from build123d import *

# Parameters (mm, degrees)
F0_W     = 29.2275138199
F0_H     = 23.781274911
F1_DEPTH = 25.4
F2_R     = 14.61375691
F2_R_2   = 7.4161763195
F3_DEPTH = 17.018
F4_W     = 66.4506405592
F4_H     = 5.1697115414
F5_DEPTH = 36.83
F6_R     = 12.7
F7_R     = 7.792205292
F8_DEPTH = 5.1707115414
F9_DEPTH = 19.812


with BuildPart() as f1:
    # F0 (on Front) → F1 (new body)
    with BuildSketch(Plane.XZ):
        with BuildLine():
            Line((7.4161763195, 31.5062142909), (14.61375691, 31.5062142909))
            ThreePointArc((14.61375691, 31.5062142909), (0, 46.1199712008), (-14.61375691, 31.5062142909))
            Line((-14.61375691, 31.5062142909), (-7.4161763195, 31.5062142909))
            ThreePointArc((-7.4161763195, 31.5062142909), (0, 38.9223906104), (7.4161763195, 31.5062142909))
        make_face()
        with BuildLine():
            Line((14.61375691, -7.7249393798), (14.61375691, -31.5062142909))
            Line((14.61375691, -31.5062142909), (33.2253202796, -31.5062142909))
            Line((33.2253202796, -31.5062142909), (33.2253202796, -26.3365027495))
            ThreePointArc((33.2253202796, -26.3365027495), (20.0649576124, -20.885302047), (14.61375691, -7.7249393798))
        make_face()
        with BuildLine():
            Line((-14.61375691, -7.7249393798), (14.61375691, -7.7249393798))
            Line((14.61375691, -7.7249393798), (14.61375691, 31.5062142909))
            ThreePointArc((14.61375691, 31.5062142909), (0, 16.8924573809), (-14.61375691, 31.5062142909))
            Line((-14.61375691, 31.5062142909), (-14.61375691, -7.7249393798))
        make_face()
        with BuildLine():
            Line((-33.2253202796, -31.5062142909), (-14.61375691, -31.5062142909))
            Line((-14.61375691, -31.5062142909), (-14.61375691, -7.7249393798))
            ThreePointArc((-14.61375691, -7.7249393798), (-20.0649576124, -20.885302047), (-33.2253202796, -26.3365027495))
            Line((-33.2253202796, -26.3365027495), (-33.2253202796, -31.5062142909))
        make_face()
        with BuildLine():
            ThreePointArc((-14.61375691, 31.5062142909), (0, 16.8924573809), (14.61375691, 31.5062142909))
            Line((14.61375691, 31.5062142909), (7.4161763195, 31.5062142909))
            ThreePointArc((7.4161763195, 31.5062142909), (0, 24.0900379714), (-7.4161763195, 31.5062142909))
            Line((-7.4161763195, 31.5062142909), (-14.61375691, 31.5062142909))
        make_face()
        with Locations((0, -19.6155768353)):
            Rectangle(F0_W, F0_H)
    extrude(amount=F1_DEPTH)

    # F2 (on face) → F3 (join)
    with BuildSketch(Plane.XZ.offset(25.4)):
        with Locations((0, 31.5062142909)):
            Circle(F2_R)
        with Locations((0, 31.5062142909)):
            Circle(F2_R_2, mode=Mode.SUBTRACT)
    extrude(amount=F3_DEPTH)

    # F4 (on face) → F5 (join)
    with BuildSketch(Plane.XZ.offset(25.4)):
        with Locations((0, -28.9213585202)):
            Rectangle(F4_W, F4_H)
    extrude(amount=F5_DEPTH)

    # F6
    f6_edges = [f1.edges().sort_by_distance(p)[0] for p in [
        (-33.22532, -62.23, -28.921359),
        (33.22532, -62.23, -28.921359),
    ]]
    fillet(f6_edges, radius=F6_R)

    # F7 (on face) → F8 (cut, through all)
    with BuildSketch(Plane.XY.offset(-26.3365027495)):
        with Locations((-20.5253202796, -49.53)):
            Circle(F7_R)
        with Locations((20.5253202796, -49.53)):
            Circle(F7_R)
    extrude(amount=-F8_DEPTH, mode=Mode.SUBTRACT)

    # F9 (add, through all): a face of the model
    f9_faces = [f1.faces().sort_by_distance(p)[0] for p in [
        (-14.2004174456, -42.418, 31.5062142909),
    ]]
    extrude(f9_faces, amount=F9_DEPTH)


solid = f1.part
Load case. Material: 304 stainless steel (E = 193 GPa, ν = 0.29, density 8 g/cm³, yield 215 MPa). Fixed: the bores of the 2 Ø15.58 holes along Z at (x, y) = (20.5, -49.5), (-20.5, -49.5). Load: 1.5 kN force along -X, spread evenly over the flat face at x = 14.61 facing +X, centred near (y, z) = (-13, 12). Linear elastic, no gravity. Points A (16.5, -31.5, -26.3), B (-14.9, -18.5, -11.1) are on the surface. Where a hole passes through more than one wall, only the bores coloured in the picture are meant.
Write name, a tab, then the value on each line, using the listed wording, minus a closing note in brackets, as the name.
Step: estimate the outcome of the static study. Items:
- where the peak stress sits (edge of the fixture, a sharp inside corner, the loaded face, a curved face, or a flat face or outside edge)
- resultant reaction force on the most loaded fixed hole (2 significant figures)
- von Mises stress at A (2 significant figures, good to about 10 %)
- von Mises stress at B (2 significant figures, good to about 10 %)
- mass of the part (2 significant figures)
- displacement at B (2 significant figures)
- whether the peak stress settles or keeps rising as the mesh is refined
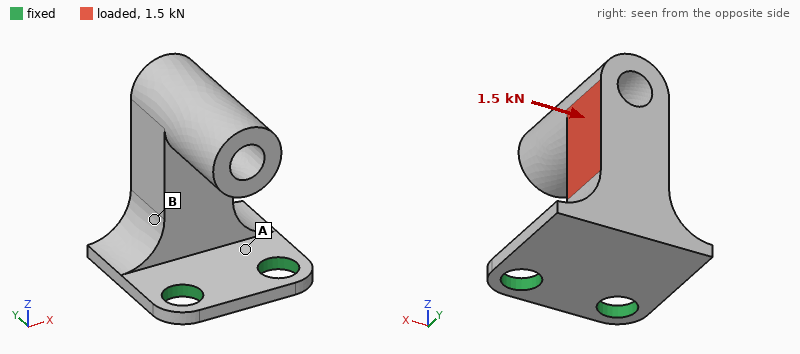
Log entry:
where the peak stress sits	edge of the fixture
resultant reaction force on the most loaded fixed hole	1.9 kN
von Mises stress at A	50 MPa
von Mises stress at B	19 MPa
mass of the part	710 g
displacement at B	28 µm
whether the peak stress settles or keeps rising as the mesh is refined	keeps rising
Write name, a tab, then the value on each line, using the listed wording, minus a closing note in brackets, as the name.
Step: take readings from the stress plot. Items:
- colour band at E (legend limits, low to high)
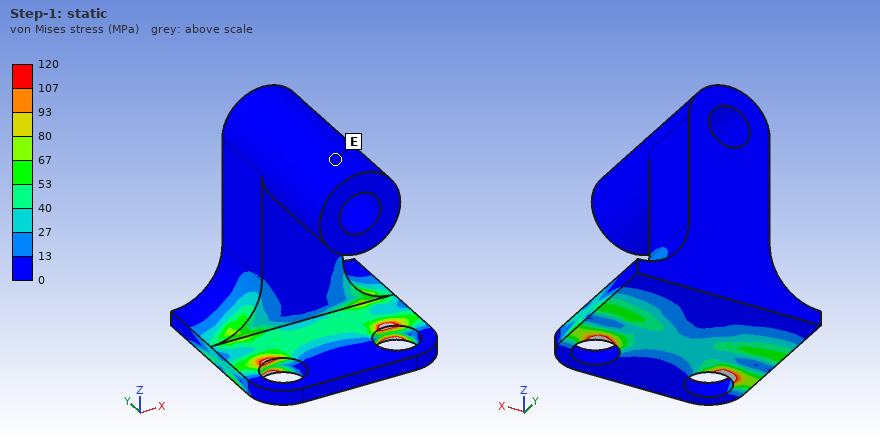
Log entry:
colour band at E	0 to 13 MPa
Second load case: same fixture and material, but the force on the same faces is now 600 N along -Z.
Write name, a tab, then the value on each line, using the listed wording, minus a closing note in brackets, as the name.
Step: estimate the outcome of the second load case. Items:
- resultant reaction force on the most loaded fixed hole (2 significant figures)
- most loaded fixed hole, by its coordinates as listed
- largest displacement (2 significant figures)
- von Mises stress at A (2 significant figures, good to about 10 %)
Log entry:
resultant reaction force on the most loaded fixed hole	500 N
most loaded fixed hole, by its coordinates as listed	(20.5, -49.5)
largest displacement	0.14 mm
von Mises stress at A	34 MPa
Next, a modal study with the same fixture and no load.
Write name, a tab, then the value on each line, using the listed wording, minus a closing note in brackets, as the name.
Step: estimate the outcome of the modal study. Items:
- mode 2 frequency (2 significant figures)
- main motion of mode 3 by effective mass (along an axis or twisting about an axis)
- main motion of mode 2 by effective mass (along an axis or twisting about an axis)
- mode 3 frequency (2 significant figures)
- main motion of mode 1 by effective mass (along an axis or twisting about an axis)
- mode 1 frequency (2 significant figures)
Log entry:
mode 2 frequency	990 Hz
main motion of mode 3 by effective mass	along Z
main motion of mode 2 by effective mass	along X
mode 3 frequency	2200 Hz
main motion of mode 1 by effective mass	along Y
mode 1 frequency	360 Hz
